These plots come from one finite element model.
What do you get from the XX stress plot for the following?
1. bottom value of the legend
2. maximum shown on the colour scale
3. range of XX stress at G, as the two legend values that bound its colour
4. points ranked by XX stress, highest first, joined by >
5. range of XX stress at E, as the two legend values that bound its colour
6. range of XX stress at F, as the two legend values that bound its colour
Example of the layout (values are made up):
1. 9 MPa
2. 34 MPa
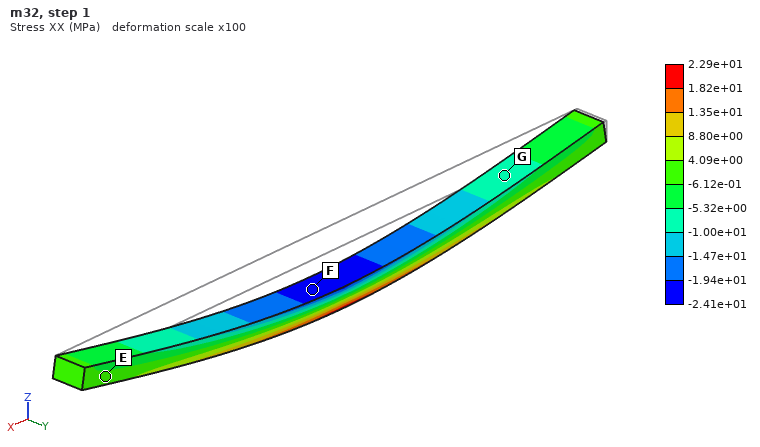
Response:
1. -2.41e+01 MPa
2. 2.29e+01 MPa
3. -1.00e+01 to -5.32e+00 MPa
4. E > G > F
5. -6.12e-01 to 4.09e+00 MPa
6. -2.41e+01 to -1.94e+01 MPa
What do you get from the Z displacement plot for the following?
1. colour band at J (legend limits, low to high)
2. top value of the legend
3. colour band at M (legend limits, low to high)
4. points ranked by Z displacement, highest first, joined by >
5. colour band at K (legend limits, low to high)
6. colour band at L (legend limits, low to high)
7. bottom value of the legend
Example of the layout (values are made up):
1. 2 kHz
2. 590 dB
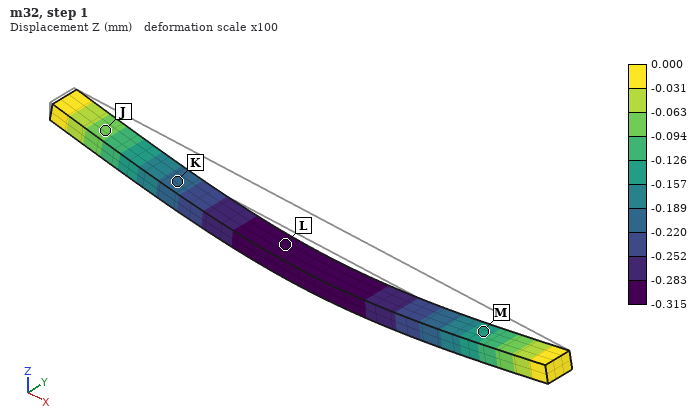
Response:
1. -0.094 to -0.063 mm
2. 0.000 mm
3. -0.157 to -0.126 mm
4. J > M > K > L
5. -0.220 to -0.189 mm
6. -0.315 to -0.283 mm
7. -0.315 mm
